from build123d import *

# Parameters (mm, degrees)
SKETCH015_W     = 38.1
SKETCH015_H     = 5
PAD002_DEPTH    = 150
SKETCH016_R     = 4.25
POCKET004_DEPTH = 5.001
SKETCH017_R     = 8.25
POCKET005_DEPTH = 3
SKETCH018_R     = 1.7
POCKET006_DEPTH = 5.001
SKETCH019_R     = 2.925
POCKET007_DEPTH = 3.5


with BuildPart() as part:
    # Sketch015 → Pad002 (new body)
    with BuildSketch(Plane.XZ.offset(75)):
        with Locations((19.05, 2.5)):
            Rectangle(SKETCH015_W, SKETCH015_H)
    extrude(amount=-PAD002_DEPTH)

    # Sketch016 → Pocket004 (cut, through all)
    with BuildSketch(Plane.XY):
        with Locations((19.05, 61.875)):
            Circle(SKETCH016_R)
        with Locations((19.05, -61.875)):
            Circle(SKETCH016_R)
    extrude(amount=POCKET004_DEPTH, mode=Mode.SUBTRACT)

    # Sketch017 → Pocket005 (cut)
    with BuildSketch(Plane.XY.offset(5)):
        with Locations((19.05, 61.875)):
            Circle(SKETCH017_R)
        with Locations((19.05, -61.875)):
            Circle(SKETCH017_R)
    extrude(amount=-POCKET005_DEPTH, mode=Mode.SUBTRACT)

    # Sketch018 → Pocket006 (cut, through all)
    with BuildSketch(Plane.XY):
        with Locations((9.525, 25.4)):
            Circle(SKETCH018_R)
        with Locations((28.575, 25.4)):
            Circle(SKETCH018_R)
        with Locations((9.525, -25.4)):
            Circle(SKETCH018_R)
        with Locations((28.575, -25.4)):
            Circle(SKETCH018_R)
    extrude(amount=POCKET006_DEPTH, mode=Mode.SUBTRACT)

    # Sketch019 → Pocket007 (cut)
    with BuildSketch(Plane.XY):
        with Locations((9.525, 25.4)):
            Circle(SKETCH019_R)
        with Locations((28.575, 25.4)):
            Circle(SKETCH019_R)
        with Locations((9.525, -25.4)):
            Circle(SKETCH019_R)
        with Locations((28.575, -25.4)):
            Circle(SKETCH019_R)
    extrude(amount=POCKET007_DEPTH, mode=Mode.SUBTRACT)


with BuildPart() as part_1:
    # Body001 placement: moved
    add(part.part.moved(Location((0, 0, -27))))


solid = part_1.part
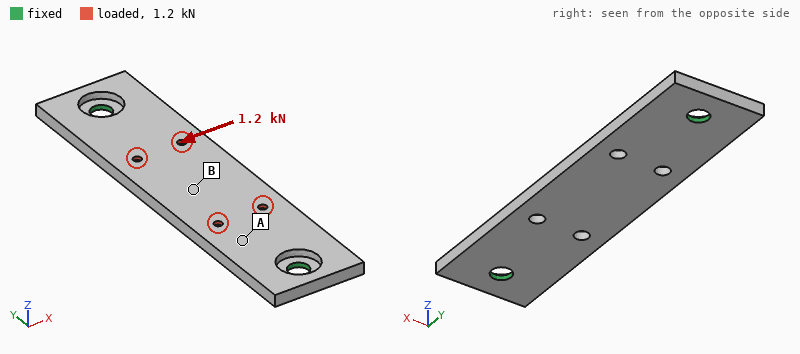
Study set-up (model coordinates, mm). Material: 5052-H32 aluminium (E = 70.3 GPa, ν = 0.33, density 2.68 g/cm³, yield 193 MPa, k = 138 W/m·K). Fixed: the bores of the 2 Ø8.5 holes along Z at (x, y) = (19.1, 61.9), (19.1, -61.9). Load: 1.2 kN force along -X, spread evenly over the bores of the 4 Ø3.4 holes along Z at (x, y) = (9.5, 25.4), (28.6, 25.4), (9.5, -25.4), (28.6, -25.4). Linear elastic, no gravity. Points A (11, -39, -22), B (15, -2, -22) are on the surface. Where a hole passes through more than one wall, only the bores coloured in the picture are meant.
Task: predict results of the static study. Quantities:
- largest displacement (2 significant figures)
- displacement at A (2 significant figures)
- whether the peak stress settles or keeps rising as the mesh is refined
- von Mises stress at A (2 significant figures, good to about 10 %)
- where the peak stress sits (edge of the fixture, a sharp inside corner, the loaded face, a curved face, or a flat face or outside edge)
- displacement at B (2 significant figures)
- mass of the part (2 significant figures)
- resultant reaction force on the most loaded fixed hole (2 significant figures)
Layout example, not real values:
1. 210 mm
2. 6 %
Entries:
1. 50 µm
2. 24 µm
3. keeps rising
4. 13 MPa
5. edge of the fixture
6. 31 µm
7. 71 g
8. 600 N
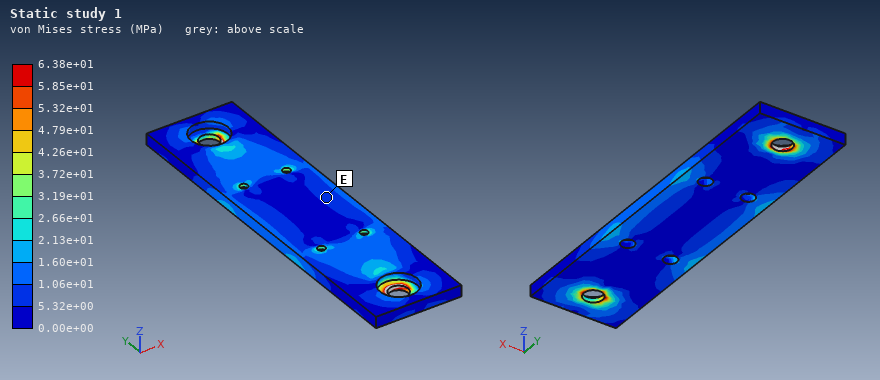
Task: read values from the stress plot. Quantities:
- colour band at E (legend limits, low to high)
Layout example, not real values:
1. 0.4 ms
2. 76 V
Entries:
1. 5.32e+00 to 1.06e+01 MPa
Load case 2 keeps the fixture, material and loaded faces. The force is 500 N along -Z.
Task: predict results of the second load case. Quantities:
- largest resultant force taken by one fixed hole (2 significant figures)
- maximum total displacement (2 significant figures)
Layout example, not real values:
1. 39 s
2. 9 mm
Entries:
1. 790 N
2. 0.17 mm
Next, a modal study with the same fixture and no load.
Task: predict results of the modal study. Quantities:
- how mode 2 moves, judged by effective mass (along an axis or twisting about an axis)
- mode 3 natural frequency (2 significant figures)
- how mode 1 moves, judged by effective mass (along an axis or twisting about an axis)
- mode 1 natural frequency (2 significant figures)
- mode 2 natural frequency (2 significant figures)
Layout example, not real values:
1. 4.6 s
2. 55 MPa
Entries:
1. twisting about Y
2. 3700 Hz
3. along Z
4. 1400 Hz
5. 2500 Hz
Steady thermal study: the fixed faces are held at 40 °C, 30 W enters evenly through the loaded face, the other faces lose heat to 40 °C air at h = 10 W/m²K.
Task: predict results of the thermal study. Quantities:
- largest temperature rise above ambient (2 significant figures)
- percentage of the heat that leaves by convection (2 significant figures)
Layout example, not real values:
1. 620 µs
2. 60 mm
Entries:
1. 31 K
2. 7.5 %
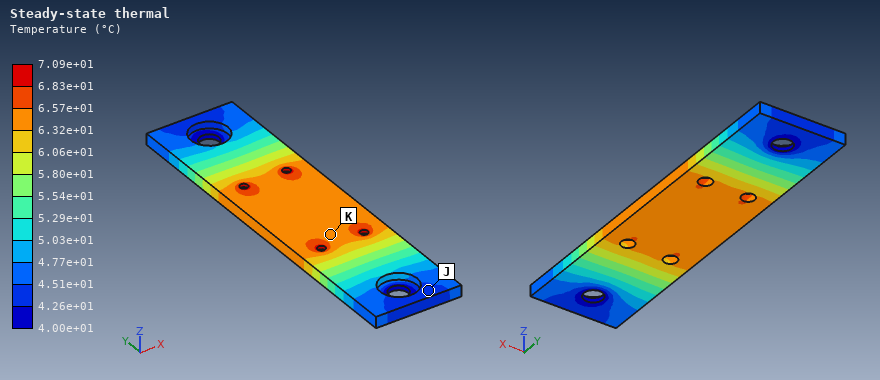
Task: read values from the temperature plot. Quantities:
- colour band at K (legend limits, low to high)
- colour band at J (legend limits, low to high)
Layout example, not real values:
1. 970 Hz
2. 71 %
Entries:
1. 6.32e+01 to 6.57e+01 °C
2. 4.26e+01 to 4.51e+01 °C
